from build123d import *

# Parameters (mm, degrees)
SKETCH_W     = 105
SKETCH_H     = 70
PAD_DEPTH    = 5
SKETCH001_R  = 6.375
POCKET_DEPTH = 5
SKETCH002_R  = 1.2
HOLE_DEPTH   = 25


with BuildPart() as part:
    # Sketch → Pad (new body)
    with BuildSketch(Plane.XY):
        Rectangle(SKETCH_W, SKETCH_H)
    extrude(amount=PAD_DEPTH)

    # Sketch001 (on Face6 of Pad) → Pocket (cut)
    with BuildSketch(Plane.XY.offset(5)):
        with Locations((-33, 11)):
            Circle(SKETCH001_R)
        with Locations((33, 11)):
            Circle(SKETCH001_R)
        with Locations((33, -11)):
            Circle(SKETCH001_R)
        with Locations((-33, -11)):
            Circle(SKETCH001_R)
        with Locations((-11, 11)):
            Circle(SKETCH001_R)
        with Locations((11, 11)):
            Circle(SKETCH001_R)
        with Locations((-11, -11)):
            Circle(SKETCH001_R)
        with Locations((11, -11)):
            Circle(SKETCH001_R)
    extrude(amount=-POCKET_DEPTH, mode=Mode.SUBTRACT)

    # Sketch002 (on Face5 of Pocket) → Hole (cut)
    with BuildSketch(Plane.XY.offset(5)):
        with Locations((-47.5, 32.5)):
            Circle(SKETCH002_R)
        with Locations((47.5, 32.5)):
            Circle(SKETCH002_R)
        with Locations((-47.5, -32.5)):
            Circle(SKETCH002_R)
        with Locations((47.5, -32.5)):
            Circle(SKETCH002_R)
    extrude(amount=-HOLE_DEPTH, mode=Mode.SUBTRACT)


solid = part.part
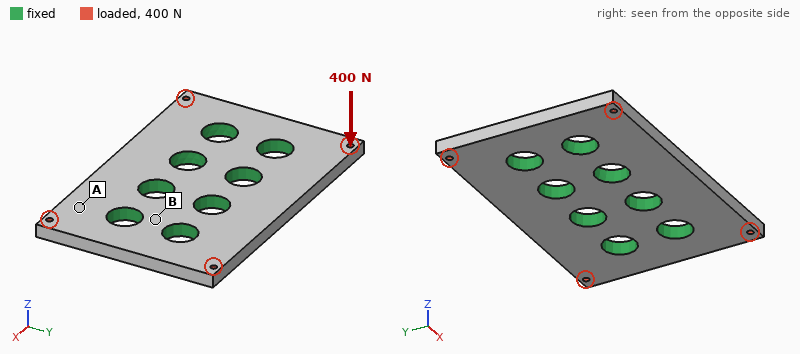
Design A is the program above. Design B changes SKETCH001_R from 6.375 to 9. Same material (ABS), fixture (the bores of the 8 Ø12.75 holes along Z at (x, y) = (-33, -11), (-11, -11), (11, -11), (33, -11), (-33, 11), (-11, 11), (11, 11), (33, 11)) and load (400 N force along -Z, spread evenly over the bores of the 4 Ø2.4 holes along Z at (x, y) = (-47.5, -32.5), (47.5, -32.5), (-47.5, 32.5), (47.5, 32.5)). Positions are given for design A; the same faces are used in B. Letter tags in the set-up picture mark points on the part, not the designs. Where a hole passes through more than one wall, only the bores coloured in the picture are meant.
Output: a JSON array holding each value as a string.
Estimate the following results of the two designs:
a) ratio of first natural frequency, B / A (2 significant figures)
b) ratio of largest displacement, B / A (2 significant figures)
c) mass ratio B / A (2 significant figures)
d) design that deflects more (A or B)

["1.3", "0.74", "0.84", "A"]
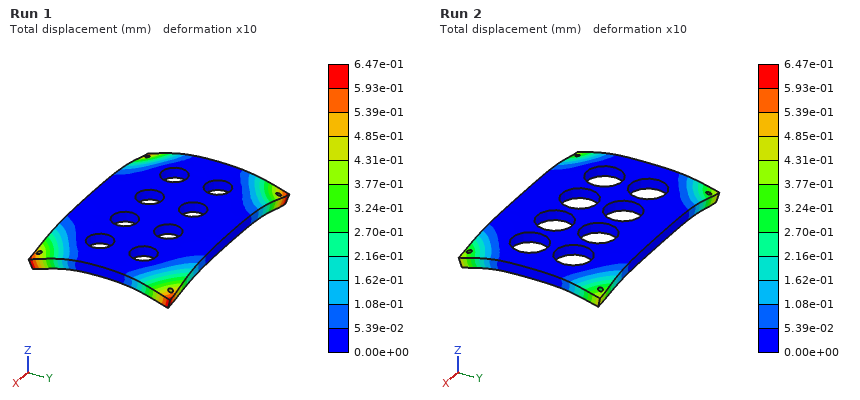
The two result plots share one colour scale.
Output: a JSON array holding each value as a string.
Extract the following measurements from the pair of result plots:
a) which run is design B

["Run 2"]
